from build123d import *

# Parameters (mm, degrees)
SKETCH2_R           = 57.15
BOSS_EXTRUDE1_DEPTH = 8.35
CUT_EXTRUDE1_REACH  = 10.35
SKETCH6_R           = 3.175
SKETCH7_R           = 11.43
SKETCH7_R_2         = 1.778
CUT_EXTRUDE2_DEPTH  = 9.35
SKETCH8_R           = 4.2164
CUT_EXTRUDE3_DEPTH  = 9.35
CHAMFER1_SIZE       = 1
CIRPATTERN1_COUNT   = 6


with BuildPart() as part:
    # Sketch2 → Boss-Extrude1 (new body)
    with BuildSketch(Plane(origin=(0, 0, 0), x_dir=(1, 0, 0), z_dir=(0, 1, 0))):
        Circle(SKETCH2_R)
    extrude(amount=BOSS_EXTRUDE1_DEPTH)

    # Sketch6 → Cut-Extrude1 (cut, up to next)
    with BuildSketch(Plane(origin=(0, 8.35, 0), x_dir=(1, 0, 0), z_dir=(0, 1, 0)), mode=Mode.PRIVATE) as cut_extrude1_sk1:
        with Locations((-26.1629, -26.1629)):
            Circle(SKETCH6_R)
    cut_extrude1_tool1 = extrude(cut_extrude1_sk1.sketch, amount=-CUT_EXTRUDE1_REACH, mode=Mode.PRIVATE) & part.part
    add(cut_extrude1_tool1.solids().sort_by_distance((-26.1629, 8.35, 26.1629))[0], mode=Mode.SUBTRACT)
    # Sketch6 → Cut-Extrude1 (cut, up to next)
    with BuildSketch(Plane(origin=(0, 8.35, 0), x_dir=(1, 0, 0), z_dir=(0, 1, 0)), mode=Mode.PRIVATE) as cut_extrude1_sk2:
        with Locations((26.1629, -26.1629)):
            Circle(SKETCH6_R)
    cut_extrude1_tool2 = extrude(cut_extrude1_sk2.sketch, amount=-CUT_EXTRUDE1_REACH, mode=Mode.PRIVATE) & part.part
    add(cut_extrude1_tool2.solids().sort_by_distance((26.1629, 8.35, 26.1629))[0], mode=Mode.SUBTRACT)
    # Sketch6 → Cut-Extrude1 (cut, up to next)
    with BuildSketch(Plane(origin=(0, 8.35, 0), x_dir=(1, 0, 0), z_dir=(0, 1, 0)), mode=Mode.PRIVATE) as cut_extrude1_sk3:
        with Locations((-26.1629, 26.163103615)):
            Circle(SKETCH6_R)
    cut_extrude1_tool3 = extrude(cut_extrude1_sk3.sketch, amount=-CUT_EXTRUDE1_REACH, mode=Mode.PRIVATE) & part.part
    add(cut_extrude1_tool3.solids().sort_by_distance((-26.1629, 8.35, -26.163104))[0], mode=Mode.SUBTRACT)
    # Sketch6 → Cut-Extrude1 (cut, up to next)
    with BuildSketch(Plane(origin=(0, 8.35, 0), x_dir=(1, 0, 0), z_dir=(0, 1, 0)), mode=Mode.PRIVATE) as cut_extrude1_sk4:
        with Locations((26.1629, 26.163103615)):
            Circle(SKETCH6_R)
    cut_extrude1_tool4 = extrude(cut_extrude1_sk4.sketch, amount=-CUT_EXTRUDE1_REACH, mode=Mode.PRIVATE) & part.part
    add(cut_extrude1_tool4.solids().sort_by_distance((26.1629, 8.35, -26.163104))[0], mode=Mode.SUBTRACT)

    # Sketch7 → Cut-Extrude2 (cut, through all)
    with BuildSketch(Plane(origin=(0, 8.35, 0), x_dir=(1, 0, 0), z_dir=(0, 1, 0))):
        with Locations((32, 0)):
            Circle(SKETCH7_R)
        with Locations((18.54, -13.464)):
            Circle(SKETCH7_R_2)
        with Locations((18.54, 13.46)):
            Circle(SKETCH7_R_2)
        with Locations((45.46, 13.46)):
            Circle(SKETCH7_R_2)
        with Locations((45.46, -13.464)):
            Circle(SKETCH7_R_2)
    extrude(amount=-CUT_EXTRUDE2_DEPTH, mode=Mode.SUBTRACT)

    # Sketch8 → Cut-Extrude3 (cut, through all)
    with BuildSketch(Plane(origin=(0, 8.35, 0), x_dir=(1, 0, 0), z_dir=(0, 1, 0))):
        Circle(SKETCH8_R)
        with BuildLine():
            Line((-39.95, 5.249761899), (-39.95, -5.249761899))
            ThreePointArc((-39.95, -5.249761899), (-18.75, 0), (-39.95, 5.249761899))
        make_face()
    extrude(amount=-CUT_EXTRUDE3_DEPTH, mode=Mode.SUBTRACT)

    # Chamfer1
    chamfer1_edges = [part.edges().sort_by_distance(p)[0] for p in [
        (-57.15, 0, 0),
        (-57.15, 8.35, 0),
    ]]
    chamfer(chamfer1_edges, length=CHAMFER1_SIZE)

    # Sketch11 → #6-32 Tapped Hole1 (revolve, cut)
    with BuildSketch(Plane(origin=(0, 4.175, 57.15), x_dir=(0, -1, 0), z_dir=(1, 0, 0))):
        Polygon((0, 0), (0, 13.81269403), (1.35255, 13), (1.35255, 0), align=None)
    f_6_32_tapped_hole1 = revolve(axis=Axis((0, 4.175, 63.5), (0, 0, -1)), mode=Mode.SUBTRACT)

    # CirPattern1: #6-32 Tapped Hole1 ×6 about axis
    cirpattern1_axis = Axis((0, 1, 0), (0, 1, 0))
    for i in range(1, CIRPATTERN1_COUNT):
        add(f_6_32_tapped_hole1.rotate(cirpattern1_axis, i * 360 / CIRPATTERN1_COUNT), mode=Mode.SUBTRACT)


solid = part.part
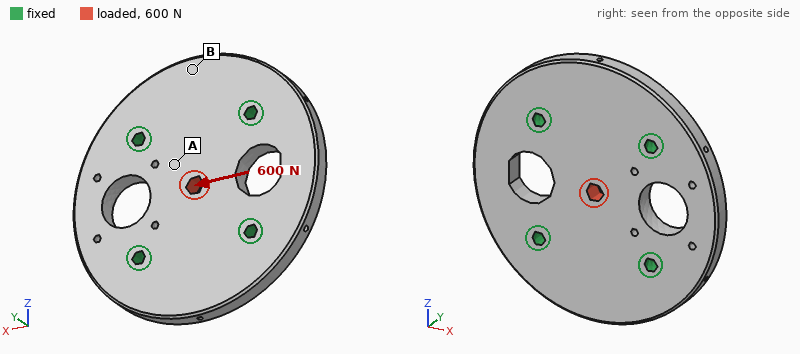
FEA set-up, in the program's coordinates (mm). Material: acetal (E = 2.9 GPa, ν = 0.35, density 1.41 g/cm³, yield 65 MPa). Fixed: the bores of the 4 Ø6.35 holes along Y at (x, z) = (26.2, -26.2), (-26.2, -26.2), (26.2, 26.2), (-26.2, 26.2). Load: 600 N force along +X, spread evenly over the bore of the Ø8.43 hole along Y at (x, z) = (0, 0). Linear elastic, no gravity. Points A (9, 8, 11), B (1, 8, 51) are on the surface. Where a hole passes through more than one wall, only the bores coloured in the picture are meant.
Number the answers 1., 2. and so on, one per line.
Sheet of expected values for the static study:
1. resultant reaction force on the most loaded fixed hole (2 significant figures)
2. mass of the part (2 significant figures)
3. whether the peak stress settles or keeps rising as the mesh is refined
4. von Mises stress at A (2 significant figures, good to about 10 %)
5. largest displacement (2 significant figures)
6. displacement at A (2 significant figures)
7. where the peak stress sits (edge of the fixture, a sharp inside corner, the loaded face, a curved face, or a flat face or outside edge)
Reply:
1. 170 N
2. 110 g
3. keeps rising
4. 1.4 MPa
5. 21 µm
6. 9.7 µm
7. a sharp inside corner
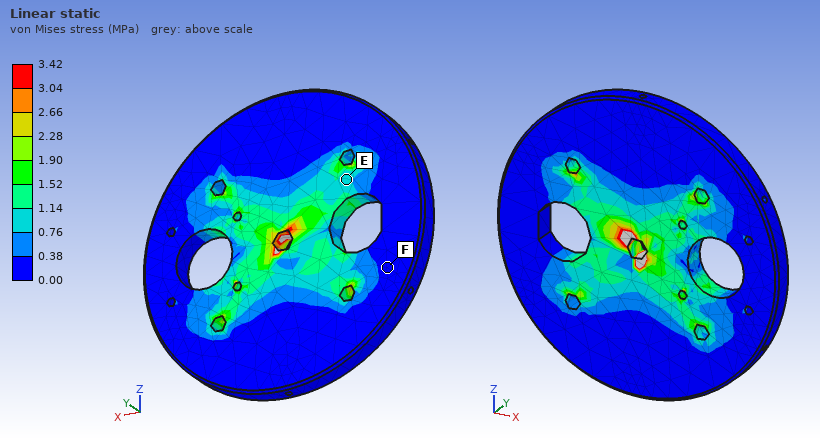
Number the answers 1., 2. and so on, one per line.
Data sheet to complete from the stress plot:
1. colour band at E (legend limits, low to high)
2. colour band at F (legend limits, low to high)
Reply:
1. 0.76 to 1.14 MPa
2. 0.00 to 0.38 MPa
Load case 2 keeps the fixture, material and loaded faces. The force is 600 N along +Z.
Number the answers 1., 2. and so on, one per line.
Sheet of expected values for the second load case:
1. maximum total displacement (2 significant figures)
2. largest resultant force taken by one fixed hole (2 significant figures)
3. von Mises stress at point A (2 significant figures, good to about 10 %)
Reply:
1. 18 µm
2. 160 N
3. 1.2 MPa
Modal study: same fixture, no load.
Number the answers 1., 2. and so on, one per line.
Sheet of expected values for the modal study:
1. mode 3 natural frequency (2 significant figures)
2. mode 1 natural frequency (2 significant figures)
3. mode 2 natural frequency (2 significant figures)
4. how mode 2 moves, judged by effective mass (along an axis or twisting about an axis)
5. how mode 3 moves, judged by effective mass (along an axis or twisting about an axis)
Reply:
1. 2000 Hz
2. 1800 Hz
3. 1900 Hz
4. twisting about Z
5. twisting about X
